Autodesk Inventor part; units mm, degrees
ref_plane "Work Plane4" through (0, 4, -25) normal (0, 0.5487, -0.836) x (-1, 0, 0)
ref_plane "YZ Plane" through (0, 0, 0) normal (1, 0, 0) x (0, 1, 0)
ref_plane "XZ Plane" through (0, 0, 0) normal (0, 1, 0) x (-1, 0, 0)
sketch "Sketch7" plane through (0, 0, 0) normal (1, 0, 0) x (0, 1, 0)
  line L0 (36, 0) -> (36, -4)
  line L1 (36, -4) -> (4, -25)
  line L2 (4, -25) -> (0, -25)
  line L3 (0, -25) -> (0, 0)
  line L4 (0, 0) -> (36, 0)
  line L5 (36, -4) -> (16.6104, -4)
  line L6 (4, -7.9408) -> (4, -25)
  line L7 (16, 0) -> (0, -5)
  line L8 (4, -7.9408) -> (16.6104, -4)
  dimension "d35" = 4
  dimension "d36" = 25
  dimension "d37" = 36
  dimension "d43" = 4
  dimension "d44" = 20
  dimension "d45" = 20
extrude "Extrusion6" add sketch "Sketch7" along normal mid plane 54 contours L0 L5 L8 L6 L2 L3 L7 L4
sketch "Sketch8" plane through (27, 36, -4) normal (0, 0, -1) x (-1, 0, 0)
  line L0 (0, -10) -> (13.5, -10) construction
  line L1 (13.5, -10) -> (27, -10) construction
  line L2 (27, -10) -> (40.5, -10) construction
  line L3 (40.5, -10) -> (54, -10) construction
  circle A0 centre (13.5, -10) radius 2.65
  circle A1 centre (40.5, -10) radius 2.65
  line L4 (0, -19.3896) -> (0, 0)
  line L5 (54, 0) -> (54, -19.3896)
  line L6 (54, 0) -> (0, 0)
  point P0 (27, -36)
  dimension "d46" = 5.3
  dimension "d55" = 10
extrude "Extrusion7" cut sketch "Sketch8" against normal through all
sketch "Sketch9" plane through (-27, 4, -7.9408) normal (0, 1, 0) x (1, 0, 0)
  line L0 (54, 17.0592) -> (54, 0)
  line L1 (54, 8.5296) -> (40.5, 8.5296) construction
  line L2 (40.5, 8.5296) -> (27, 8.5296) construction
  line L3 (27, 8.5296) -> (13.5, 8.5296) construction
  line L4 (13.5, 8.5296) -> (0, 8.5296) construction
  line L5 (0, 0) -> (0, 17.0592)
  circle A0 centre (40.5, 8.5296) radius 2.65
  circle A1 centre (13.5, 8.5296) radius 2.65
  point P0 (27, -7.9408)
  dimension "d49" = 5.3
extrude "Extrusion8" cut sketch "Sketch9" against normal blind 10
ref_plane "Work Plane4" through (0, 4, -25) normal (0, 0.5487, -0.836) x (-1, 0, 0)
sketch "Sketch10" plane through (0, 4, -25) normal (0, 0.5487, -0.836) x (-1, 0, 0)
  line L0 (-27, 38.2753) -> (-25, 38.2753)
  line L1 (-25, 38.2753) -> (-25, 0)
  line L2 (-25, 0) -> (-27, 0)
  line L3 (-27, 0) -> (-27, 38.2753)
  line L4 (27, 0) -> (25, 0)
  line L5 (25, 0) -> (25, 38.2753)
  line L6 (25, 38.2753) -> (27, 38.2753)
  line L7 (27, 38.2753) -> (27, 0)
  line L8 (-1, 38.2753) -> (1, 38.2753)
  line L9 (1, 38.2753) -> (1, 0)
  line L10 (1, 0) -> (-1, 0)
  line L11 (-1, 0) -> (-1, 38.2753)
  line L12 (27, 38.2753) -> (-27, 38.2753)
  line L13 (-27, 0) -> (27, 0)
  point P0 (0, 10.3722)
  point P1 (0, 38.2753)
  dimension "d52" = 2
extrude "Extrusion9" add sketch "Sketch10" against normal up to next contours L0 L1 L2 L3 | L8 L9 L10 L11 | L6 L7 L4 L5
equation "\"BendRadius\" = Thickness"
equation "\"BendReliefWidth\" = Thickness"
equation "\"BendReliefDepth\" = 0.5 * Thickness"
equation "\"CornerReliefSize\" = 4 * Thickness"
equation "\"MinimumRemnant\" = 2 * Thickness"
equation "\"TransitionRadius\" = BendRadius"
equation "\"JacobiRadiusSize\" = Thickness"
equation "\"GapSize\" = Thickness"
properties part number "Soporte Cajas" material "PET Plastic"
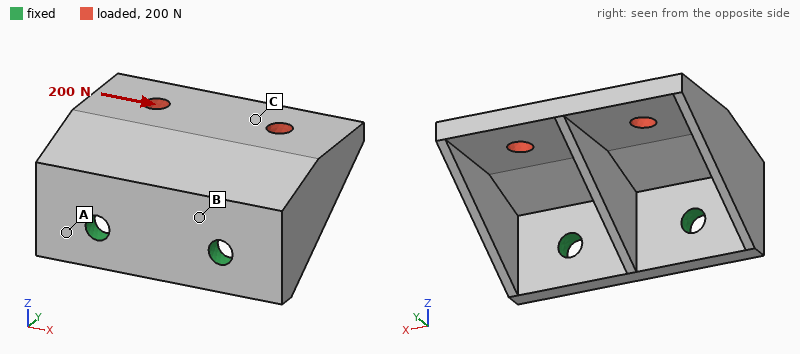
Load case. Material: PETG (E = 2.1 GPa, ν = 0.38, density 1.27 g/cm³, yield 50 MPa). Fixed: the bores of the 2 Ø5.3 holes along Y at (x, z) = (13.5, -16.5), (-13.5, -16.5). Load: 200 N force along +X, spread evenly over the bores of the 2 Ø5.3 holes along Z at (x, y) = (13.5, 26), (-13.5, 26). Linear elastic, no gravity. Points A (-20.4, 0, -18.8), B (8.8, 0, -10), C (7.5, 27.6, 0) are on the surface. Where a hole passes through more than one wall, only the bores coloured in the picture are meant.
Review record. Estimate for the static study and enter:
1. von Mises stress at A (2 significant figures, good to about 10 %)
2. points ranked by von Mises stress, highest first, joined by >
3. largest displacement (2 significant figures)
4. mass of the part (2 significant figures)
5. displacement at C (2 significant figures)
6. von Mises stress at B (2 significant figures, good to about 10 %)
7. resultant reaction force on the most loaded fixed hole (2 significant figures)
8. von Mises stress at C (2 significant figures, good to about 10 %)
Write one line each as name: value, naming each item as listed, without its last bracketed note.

von Mises stress at A: 6.9 MPa
points ranked by von Mises stress, highest first, joined by >: A > B > C
largest displacement: 0.70 mm
mass of the part: 17 g
displacement at C: 0.31 mm
von Mises stress at B: 4.2 MPa
resultant reaction force on the most loaded fixed hole: 200 N
von Mises stress at C: 1.9 MPa
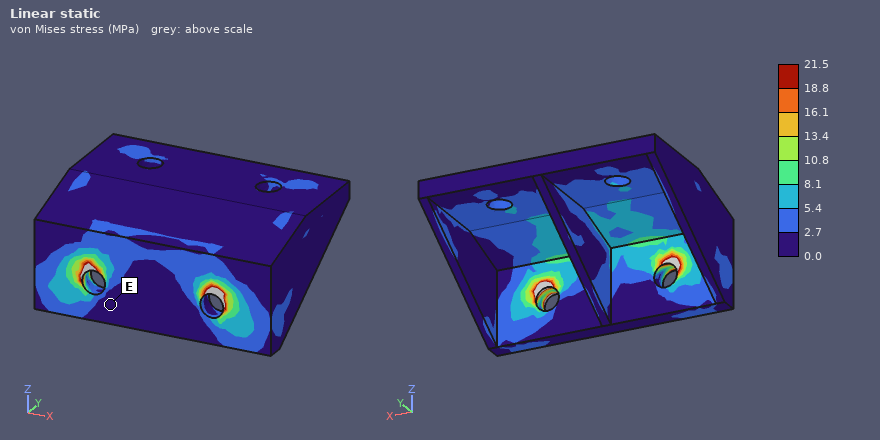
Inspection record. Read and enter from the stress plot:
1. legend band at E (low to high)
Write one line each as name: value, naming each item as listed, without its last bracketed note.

legend band at E: 0.0 to 2.7 MPa
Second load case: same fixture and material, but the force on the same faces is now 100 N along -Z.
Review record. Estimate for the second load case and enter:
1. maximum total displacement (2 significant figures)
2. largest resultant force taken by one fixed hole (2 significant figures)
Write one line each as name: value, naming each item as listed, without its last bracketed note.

maximum total displacement: 0.71 mm
largest resultant force taken by one fixed hole: 50 N
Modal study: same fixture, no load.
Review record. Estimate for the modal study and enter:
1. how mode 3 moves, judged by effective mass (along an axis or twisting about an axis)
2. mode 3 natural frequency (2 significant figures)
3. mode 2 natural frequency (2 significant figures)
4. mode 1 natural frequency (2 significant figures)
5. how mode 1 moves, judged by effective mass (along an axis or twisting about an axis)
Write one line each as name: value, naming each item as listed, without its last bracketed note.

how mode 3 moves, judged by effective mass: along X
mode 3 natural frequency: 2000 Hz
mode 2 natural frequency: 960 Hz
mode 1 natural frequency: 800 Hz
how mode 1 moves, judged by effective mass: along Z
